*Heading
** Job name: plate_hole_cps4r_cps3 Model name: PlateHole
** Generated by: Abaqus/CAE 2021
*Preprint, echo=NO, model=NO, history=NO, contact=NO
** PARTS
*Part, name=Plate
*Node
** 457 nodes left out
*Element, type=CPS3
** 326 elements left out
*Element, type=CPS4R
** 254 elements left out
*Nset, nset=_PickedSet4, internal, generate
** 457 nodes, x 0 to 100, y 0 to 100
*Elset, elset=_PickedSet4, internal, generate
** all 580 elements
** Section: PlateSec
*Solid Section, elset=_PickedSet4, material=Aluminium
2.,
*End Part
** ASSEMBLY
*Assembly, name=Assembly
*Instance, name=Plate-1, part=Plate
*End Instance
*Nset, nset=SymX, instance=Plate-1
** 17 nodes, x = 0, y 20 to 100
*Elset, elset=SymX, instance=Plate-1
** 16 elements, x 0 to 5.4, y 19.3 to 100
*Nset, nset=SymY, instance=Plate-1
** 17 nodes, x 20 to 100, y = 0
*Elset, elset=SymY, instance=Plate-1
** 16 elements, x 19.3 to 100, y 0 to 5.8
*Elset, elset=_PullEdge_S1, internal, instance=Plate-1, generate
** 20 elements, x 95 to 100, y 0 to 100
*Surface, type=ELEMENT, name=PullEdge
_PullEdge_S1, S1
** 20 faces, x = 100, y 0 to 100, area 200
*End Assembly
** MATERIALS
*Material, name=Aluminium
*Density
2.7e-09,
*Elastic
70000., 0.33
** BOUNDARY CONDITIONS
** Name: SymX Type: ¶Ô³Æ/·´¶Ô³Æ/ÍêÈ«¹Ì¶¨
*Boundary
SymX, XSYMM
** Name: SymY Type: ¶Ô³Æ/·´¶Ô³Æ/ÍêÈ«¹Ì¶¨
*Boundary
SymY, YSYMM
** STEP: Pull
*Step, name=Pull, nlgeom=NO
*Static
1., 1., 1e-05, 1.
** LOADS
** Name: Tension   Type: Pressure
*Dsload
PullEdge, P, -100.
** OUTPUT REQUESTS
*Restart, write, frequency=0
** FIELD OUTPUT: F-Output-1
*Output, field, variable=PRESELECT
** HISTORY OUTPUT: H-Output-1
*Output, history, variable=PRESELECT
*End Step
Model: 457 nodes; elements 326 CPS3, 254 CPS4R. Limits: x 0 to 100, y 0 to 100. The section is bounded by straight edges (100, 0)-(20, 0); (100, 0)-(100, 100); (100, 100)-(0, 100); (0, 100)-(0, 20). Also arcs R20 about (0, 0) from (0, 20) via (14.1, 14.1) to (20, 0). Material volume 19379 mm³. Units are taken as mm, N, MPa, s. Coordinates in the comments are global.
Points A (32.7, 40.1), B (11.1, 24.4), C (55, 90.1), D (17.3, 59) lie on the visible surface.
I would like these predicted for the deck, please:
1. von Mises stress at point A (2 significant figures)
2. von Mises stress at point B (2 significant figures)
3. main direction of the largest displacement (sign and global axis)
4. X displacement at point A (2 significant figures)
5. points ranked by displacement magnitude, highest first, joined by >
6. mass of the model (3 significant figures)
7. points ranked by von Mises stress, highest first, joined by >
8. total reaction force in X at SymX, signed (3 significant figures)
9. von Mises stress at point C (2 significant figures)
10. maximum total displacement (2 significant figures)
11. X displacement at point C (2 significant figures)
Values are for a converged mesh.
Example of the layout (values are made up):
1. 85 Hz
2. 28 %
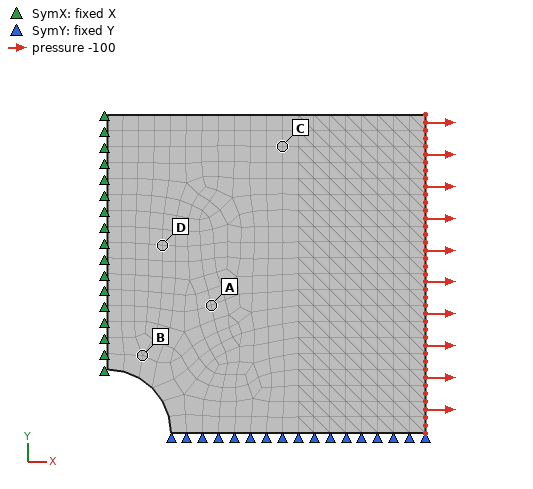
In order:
1. 130 MPa
2. 170 MPa
3. +X
4. 0.060 mm
5. C > A > D > B
6. 0.0523 kg
7. B > A > D > C
8. -20000 N
9. 100 MPa
10. 0.17 mm
11. 0.076 mm
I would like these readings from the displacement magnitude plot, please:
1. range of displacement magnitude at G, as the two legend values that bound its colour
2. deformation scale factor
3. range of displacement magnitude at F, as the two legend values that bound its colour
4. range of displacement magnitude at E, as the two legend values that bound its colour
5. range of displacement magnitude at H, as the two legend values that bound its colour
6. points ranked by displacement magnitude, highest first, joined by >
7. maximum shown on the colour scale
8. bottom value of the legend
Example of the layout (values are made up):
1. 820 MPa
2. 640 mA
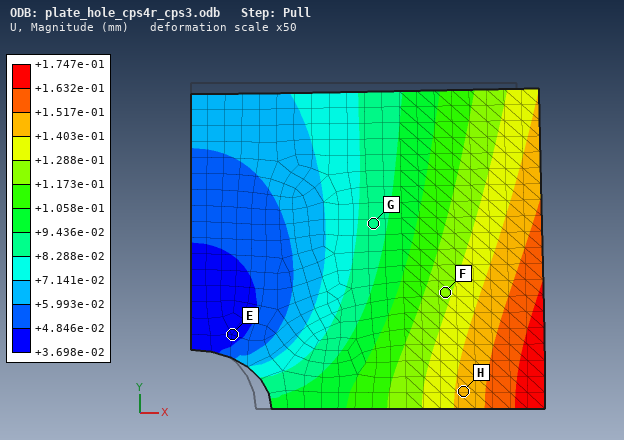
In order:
1. +8.288e-02 to +9.436e-02 mm
2. 50
3. +1.173e-01 to +1.288e-01 mm
4. +3.698e-02 to +4.846e-02 mm
5. +1.403e-01 to +1.517e-01 mm
6. H > F > G > E
7. +1.747e-01 mm
8. +3.698e-02 mm
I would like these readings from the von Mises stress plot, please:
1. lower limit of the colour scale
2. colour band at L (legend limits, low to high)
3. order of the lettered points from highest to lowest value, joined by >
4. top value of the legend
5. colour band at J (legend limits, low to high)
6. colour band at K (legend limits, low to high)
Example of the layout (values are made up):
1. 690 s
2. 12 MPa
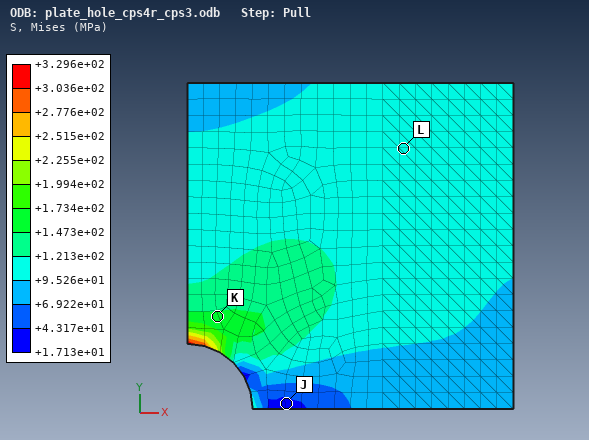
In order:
1. +1.713e+01 MPa
2. +9.526e+01 to +1.213e+02 MPa
3. K > L > J
4. +3.296e+02 MPa
5. +1.713e+01 to +4.317e+01 MPa
6. +1.473e+02 to +1.734e+02 MPa
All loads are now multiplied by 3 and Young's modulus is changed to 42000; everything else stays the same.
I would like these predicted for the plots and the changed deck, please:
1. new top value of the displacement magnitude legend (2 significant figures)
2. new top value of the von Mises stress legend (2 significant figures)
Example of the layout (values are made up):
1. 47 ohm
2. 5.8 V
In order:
1. 0.87 mm
2. 990 MPa
